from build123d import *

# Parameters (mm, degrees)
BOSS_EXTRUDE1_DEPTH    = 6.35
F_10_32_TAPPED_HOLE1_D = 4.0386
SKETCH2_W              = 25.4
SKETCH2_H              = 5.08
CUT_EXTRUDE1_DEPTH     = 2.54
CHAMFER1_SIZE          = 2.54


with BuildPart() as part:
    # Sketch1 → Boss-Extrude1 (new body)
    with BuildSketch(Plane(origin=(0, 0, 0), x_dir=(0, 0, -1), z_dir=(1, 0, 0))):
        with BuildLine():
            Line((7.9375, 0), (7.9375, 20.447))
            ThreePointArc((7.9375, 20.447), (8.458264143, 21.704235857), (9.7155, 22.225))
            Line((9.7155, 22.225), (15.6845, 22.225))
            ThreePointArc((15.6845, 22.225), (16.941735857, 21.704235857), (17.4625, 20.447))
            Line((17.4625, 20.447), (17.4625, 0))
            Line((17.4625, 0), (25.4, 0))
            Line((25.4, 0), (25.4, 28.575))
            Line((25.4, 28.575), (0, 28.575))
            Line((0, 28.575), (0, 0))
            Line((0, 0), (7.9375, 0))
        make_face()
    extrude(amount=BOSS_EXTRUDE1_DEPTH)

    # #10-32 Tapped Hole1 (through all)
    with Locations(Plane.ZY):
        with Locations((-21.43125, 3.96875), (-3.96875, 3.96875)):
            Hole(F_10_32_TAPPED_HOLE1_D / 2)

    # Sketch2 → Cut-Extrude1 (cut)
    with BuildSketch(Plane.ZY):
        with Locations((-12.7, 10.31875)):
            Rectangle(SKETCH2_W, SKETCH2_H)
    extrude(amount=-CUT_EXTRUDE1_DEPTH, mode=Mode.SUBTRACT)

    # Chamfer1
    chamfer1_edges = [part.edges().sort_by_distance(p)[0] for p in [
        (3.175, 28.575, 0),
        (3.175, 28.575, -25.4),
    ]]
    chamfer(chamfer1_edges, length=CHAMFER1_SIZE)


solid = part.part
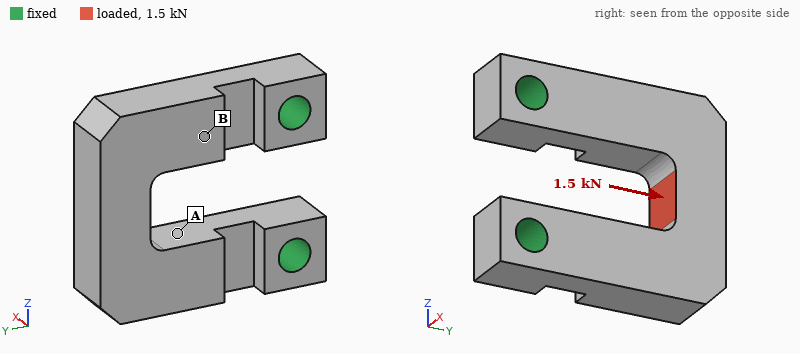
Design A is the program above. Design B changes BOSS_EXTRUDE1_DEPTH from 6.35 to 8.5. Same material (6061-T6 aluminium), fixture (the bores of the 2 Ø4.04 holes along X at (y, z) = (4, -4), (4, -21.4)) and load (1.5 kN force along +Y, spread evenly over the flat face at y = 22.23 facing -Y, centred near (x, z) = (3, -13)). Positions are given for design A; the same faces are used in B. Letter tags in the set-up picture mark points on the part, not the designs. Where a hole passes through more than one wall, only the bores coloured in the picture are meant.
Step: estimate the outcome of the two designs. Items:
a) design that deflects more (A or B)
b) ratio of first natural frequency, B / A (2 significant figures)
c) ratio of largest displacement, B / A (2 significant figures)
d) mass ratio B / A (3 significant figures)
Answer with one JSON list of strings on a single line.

["A", "1.5", "0.36", "1.36"]
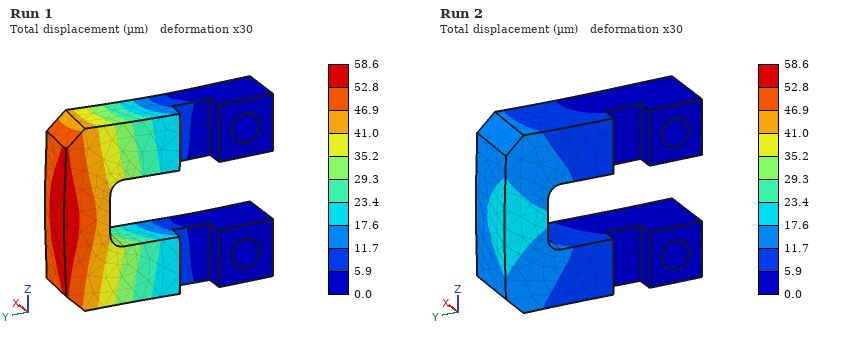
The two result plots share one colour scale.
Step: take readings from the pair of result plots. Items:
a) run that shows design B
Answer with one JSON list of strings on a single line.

["Run 2"]
